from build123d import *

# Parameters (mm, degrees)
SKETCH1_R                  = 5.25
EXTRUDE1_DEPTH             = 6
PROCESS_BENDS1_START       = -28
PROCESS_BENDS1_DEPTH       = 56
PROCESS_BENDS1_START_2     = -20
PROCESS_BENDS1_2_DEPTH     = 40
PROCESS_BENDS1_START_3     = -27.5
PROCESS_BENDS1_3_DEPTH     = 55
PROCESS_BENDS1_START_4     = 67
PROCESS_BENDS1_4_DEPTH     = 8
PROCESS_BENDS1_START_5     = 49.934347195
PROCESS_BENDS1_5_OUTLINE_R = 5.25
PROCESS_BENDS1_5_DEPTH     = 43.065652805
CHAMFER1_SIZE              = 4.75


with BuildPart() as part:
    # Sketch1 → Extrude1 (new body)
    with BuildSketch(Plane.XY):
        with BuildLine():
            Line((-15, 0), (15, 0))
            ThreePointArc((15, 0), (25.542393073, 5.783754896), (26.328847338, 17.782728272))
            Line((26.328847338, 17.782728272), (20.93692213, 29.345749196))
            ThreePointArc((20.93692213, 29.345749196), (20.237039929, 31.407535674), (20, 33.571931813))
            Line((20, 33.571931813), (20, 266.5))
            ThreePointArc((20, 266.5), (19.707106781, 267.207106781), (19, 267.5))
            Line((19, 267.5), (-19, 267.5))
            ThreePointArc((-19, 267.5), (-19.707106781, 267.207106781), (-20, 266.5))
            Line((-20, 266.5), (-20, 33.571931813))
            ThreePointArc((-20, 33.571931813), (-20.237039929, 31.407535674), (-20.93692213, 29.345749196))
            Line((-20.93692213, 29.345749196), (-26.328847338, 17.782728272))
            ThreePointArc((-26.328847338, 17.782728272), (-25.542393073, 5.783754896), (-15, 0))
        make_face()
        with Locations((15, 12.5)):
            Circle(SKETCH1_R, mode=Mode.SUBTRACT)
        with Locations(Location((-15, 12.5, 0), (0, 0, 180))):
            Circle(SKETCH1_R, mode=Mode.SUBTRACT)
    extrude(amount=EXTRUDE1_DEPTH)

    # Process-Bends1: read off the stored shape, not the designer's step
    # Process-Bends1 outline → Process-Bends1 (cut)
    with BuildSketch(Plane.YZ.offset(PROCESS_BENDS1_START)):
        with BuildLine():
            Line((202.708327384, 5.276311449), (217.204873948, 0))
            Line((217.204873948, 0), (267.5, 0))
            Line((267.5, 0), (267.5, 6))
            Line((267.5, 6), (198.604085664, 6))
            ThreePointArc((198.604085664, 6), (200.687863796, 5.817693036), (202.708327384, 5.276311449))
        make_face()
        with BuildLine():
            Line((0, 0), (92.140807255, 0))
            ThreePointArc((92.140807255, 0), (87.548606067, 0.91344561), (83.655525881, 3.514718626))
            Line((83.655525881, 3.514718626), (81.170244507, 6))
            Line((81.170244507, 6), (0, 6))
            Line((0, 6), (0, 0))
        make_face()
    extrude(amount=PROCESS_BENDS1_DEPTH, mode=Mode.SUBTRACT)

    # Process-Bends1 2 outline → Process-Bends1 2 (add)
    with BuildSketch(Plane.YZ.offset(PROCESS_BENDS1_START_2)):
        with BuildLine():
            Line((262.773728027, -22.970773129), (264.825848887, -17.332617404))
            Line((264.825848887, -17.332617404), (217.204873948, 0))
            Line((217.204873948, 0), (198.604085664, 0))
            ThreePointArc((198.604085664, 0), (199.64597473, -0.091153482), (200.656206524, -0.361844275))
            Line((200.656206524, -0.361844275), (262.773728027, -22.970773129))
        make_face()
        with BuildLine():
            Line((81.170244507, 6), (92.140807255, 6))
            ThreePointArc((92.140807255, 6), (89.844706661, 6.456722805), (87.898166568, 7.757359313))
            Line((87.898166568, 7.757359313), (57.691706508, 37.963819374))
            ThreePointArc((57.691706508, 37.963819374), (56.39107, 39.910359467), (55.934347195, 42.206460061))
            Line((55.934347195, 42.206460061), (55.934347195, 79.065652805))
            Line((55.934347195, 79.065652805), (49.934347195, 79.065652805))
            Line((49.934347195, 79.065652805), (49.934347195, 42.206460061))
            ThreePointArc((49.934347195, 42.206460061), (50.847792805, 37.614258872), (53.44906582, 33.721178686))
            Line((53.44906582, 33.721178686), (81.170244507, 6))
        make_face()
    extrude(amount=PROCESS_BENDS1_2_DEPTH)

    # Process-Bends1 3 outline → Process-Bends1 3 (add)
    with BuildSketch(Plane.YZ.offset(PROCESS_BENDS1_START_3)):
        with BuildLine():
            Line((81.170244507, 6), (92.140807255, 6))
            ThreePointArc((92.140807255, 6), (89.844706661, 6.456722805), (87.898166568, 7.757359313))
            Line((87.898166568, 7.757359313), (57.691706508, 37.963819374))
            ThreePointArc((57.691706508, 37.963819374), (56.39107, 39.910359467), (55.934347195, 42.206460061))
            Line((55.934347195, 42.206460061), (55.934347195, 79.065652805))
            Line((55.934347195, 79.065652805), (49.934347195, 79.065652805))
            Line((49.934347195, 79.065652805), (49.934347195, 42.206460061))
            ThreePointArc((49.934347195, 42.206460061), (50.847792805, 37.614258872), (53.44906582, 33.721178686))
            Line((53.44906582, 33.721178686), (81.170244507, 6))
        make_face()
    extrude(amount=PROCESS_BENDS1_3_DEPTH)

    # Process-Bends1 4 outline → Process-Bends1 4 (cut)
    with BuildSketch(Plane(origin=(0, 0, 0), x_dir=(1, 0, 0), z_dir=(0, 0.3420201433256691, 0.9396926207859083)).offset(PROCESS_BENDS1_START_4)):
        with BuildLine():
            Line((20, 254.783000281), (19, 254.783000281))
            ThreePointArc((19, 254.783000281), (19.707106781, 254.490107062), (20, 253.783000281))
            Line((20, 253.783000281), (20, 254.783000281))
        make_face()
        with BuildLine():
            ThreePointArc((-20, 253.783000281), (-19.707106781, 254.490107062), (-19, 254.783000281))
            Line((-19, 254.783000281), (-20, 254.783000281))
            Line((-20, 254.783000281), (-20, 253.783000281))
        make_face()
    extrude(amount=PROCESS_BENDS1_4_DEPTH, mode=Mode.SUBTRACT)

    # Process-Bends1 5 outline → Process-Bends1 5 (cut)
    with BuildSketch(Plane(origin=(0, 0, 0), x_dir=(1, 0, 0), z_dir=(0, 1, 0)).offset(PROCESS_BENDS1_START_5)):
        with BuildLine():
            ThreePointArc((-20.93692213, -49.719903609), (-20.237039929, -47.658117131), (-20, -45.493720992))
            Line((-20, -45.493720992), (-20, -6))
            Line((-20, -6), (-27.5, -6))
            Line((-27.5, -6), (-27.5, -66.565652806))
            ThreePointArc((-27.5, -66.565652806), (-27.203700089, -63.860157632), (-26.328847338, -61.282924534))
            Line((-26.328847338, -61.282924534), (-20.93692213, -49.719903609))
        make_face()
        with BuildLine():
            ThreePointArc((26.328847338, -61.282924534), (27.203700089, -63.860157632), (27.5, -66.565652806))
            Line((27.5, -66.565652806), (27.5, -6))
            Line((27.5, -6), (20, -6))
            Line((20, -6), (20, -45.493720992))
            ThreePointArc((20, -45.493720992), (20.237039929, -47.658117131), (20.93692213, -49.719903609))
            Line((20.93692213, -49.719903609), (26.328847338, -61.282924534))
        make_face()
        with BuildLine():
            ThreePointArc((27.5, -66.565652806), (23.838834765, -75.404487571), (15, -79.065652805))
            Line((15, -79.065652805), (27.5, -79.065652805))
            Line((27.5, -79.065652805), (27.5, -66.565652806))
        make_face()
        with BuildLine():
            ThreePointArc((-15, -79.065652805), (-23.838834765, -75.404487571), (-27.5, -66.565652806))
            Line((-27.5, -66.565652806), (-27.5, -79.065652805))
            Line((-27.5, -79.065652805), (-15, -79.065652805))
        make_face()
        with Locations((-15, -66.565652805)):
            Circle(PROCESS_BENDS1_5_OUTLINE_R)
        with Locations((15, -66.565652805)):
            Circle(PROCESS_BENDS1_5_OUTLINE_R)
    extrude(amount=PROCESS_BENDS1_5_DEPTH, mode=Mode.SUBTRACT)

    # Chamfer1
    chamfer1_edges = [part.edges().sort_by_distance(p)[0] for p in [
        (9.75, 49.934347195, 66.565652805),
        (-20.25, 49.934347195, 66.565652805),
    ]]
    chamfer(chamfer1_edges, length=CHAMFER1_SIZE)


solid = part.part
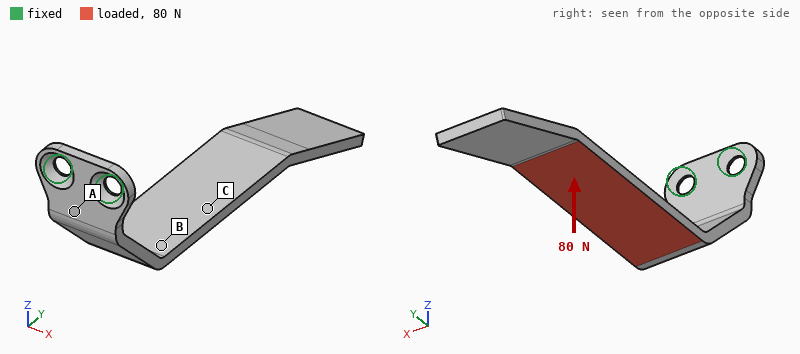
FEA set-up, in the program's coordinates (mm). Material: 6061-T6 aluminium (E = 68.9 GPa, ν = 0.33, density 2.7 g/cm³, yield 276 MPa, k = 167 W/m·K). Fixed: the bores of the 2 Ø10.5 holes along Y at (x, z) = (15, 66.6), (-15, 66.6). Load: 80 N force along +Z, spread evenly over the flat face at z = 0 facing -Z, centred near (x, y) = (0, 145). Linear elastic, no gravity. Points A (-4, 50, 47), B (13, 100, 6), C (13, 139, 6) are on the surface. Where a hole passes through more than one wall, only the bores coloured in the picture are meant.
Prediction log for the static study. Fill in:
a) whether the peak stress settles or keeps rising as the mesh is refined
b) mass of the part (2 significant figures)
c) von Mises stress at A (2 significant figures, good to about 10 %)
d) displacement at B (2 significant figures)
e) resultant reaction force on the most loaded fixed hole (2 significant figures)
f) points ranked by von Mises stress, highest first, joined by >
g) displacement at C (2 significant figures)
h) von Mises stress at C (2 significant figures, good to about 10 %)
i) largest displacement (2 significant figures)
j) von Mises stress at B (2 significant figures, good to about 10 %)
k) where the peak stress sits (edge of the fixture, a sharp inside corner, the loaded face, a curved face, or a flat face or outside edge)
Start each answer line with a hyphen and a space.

- keeps rising
- 170 g
- 28 MPa
- 0.54 mm
- 130 N
- A > B > C
- 0.98 mm
- 5.8 MPa
- 2.8 mm
- 15 MPa
- edge of the fixture
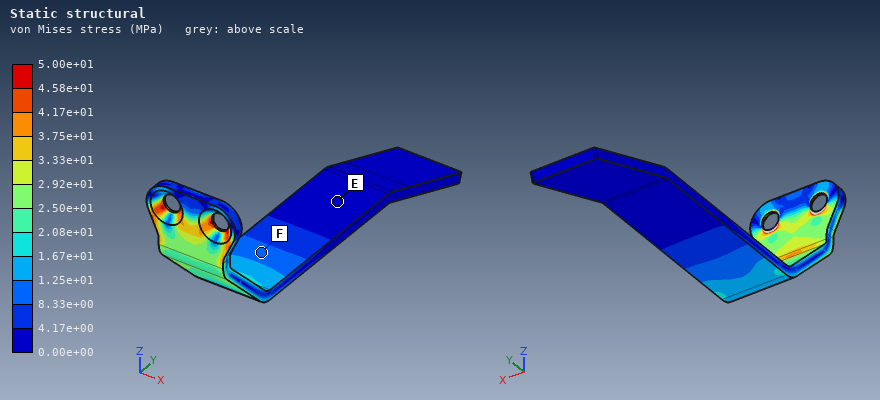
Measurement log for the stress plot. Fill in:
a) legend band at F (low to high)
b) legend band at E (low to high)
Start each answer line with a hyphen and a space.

- 8.33e+00 to 1.25e+01 MPa
- 0.00e+00 to 4.17e+00 MPa
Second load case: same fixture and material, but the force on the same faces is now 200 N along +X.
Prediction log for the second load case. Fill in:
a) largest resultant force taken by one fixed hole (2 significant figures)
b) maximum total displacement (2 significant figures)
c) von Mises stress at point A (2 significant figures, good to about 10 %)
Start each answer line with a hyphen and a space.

- 610 N
- 1.8 mm
- 56 MPa
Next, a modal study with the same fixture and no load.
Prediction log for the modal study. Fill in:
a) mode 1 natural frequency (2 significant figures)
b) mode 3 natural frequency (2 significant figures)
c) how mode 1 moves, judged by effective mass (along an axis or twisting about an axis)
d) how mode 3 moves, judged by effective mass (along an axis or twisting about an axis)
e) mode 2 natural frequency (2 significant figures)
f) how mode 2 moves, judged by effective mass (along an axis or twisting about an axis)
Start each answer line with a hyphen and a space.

- 76 Hz
- 400 Hz
- along Z
- along Y
- 160 Hz
- along X
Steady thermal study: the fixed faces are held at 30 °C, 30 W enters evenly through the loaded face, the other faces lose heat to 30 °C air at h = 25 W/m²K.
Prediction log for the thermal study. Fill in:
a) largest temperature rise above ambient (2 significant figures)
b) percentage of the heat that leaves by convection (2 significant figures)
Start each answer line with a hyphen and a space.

- 47 K
- 52 %
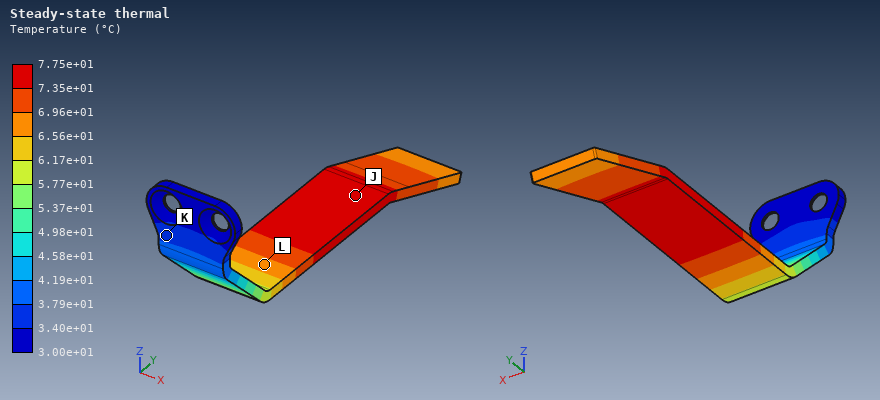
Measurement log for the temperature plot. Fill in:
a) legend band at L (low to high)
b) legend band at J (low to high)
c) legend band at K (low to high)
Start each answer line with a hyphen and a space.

- 6.56e+01 to 6.96e+01 °C
- 7.35e+01 to 7.75e+01 °C
- 3.40e+01 to 3.79e+01 °C
